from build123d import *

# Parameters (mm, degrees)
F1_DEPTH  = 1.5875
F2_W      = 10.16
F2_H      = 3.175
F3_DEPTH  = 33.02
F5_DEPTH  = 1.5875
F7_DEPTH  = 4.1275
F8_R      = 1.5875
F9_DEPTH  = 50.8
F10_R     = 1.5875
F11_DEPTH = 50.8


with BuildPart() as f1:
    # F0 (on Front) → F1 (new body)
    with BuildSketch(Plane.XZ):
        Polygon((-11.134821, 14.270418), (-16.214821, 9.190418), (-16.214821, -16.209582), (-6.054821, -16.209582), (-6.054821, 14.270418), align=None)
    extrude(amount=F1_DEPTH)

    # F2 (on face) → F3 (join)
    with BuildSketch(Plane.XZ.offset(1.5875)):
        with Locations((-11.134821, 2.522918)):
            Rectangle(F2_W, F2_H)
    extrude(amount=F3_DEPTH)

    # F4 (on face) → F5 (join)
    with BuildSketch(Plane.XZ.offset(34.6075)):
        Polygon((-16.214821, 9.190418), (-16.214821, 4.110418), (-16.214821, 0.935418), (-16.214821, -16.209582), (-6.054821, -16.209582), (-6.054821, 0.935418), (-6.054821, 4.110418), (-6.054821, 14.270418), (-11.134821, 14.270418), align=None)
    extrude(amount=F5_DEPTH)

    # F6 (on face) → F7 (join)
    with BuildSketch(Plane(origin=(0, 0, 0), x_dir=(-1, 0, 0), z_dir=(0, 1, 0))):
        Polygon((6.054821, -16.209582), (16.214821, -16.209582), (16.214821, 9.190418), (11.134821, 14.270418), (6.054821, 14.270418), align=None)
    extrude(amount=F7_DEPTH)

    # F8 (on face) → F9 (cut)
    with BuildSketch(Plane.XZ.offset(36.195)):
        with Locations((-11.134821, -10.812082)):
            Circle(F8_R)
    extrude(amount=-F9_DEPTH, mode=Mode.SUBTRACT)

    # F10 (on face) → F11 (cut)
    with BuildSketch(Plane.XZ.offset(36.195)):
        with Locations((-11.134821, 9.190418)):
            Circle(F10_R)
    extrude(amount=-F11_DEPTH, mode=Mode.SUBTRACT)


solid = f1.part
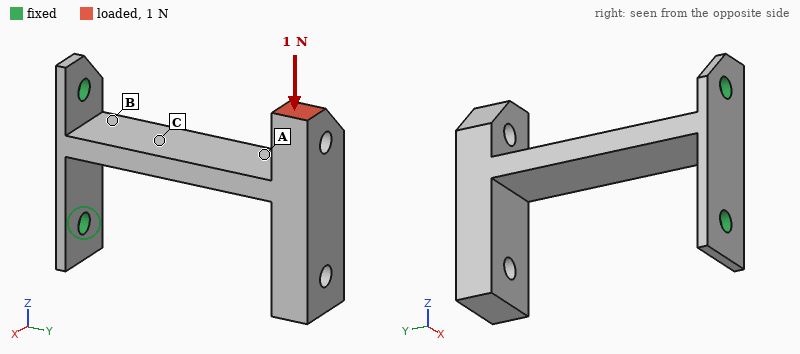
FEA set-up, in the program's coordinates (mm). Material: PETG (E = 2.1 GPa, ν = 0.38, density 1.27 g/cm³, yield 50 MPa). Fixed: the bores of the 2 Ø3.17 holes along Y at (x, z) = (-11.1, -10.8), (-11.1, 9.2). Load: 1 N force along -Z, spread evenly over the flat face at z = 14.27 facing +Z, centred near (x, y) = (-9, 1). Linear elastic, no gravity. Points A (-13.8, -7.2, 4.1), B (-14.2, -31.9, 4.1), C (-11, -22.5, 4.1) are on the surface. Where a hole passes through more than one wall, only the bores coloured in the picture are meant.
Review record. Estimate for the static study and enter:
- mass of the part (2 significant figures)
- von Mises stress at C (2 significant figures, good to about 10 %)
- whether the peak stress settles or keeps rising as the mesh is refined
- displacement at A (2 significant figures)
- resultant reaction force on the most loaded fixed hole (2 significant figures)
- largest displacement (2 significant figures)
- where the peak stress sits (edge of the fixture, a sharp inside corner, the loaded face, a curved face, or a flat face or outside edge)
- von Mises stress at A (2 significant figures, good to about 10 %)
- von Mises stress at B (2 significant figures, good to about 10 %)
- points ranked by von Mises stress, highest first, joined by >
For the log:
4.0 g
1.4 MPa
keeps rising
0.32 mm
2.6 N
0.60 mm
edge of the fixture
0.51 MPa
1.9 MPa
B > C > A
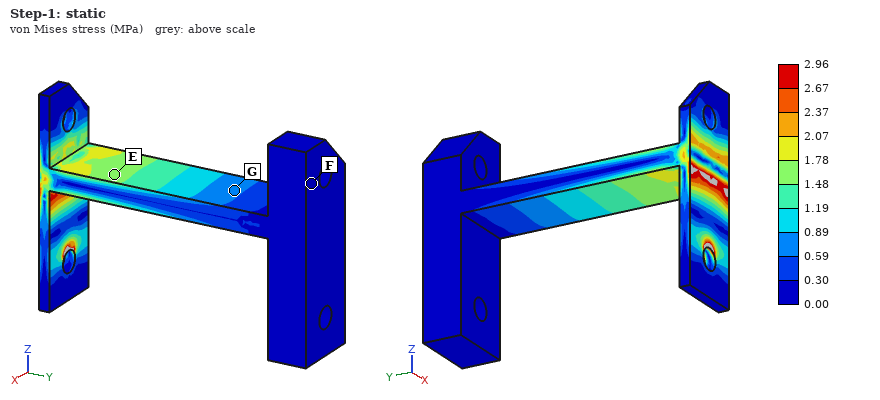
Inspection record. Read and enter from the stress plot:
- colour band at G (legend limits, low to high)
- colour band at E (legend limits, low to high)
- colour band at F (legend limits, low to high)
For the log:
0.59 to 0.89 MPa
1.48 to 1.78 MPa
0.00 to 0.30 MPa
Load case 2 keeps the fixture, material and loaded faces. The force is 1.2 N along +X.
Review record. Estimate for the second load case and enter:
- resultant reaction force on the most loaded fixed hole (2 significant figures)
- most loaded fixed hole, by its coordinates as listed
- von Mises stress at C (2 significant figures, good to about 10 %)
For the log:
1.7 N
(-11.1, 9.2)
0.99 MPa
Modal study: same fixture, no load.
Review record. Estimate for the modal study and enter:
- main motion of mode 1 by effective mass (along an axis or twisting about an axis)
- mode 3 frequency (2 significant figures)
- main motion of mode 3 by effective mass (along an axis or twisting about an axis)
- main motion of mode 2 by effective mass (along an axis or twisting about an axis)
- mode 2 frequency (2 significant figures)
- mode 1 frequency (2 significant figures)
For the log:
along Z
550 Hz
twisting about Y
along X
180 Hz
150 Hz
